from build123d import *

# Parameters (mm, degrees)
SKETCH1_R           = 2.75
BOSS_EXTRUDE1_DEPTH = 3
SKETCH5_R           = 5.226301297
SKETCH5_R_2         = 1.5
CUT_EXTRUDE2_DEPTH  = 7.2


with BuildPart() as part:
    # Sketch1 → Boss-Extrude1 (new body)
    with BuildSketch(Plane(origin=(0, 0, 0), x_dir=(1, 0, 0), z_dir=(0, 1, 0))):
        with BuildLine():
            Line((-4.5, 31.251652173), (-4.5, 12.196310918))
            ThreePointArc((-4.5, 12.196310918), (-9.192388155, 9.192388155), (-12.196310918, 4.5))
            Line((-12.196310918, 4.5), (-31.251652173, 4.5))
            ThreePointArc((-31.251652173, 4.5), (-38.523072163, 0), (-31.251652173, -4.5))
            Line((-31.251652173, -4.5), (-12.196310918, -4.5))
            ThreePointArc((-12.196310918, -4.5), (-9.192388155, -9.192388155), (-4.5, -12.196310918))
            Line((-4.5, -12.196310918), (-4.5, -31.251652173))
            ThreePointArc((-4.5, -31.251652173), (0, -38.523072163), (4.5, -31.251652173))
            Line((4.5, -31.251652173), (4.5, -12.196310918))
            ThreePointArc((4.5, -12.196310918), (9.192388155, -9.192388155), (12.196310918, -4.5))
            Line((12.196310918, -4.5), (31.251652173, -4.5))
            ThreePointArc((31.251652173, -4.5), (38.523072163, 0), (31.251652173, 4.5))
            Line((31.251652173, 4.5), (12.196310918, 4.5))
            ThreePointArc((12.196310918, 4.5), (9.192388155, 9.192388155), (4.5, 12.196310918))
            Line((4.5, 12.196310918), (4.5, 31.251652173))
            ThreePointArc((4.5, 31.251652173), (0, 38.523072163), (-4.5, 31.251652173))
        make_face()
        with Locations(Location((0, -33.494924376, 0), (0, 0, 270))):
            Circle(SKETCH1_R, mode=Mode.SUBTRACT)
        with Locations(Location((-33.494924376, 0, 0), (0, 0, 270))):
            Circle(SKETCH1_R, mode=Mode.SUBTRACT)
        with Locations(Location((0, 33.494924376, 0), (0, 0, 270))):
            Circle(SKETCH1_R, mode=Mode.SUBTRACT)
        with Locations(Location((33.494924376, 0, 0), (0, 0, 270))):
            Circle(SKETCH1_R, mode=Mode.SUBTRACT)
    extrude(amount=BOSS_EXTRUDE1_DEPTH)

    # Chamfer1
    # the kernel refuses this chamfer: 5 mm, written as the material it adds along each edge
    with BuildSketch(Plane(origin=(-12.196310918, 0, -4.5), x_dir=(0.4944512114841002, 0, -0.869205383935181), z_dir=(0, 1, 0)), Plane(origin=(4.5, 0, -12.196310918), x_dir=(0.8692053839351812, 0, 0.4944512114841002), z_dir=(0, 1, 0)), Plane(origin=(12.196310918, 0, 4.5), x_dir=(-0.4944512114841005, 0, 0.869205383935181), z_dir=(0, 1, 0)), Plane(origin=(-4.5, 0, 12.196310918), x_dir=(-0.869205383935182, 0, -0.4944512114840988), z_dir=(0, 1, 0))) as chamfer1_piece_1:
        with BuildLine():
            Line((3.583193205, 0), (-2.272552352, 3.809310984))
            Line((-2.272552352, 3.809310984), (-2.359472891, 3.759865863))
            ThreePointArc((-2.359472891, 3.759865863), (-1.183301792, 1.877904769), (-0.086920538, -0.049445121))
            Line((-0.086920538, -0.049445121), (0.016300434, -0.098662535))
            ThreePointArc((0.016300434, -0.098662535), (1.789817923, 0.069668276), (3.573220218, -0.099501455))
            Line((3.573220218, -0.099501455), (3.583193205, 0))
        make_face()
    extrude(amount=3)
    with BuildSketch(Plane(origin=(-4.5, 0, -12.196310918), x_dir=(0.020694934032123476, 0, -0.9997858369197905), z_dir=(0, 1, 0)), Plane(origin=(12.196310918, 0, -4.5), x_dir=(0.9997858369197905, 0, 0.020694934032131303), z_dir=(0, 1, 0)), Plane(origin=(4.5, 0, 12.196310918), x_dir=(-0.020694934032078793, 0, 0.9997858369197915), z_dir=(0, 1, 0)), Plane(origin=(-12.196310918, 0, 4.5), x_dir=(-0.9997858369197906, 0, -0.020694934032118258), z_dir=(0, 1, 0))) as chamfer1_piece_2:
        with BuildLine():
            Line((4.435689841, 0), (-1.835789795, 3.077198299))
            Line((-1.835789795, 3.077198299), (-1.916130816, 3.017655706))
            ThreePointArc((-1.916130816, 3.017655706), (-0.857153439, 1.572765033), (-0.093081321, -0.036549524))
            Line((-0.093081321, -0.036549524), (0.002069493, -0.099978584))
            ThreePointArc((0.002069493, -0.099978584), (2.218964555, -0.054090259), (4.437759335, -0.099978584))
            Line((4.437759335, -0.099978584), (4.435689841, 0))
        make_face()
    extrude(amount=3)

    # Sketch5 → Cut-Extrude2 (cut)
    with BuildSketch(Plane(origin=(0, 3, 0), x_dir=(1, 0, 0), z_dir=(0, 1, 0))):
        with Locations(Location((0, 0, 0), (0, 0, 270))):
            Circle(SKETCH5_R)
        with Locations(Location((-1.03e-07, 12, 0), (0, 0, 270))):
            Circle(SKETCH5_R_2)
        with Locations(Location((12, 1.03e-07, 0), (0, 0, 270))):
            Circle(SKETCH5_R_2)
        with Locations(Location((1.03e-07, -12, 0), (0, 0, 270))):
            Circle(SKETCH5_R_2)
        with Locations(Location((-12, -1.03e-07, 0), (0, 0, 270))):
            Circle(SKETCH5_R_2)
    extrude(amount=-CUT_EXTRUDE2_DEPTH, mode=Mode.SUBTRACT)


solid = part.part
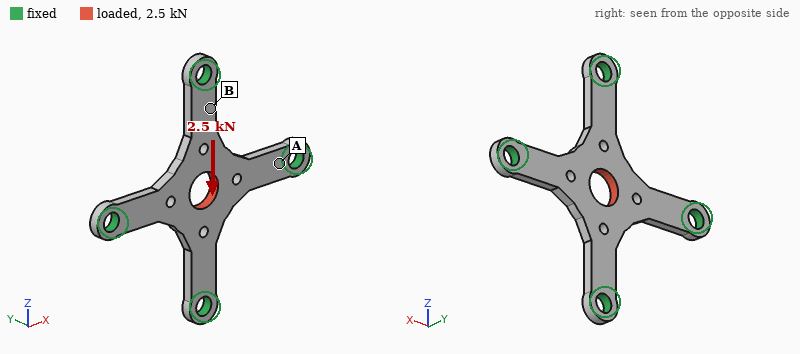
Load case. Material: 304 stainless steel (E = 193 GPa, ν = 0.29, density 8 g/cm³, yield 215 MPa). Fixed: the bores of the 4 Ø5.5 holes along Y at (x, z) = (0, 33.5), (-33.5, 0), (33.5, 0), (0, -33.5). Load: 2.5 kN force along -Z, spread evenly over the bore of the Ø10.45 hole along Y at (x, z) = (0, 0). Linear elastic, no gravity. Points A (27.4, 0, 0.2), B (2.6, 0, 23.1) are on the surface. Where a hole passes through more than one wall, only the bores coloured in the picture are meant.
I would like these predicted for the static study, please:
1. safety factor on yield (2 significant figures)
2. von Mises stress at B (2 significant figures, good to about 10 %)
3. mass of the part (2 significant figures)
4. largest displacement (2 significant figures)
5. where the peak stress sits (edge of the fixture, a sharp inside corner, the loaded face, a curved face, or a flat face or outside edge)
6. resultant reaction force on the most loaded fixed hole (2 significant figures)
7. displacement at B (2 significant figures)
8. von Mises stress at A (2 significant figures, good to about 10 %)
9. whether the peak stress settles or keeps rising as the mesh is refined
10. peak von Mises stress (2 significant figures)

2.0
42 MPa
31 g
6.3 µm
a curved face
1.1 kN
1.9 µm
11 MPa
settles
110 MPa
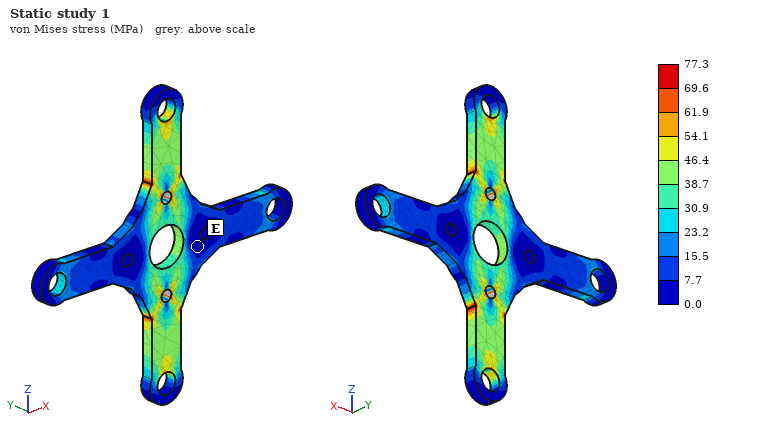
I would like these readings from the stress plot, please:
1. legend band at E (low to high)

0.0 to 7.7 MPa
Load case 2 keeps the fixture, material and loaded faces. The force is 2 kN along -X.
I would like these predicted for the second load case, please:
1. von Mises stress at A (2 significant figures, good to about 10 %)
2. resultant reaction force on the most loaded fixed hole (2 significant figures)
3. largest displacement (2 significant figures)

39 MPa
910 N
5.1 µm
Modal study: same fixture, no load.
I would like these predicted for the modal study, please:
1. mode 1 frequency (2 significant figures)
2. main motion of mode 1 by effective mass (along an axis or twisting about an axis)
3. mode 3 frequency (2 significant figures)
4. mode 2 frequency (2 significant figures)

4500 Hz
along Y
9800 Hz
9800 Hz
